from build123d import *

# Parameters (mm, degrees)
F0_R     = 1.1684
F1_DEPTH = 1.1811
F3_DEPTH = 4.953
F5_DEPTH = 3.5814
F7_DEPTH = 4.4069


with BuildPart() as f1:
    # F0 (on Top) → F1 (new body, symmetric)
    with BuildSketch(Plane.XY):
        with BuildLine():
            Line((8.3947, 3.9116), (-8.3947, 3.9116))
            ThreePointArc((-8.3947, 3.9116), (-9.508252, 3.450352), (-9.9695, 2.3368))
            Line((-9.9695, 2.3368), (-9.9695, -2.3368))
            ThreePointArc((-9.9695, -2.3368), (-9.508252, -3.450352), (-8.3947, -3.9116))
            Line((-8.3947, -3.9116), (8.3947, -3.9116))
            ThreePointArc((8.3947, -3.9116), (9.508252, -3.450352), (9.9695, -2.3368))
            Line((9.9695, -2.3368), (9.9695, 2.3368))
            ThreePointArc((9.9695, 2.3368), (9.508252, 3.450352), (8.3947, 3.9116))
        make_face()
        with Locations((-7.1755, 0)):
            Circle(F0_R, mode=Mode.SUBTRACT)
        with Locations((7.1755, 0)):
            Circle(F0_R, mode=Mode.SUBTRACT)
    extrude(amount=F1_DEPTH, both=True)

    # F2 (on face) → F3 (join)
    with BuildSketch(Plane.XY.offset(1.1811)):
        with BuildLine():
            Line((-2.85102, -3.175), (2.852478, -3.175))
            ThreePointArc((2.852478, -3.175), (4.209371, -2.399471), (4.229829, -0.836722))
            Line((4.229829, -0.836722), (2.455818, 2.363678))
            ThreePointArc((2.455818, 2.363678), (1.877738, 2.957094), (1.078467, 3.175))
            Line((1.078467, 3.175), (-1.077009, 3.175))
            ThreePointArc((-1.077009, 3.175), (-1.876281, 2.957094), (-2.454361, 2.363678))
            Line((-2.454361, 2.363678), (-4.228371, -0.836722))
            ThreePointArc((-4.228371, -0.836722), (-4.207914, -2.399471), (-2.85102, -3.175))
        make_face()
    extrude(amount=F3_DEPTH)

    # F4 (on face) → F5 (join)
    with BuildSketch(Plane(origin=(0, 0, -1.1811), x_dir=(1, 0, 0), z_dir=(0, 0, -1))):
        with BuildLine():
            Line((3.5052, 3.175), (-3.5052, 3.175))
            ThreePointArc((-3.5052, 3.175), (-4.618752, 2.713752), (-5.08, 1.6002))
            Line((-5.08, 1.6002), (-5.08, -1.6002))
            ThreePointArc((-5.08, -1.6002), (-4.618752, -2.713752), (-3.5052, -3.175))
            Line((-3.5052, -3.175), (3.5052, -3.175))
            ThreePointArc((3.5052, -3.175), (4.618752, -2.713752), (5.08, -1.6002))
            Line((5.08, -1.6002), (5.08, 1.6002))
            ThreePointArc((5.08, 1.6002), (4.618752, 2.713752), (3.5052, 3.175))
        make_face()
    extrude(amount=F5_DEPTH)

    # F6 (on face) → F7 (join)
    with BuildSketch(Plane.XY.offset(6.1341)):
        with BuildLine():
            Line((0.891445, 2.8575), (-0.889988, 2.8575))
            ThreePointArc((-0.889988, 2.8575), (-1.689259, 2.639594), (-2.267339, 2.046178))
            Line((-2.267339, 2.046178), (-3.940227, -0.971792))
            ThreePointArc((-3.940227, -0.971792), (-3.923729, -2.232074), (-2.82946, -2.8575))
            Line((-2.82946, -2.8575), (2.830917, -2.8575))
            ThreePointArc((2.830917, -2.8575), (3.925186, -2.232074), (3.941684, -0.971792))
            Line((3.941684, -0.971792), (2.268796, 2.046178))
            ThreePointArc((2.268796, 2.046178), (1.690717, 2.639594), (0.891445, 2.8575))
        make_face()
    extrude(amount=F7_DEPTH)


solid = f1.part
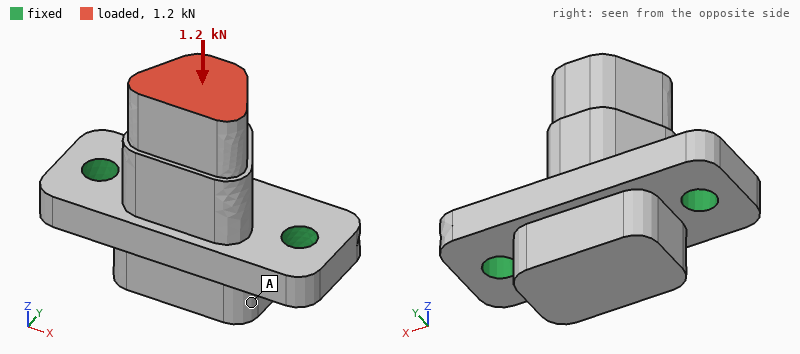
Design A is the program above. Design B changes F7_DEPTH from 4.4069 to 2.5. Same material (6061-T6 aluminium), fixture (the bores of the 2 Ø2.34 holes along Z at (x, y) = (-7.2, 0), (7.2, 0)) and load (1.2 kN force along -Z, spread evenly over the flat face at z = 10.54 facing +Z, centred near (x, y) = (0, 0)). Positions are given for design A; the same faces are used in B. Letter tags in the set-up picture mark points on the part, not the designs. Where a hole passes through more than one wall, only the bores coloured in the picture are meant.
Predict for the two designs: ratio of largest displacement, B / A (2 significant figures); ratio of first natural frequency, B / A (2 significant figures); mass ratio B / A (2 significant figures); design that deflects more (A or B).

0.92
1.3
0.93
A
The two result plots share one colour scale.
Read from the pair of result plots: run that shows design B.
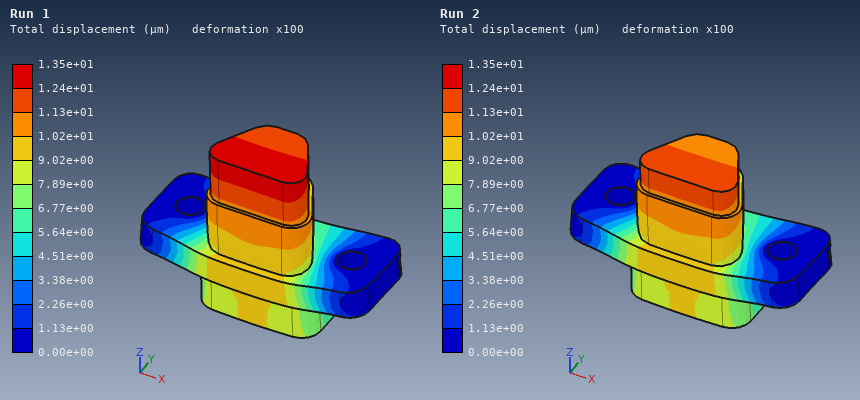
Run 2
